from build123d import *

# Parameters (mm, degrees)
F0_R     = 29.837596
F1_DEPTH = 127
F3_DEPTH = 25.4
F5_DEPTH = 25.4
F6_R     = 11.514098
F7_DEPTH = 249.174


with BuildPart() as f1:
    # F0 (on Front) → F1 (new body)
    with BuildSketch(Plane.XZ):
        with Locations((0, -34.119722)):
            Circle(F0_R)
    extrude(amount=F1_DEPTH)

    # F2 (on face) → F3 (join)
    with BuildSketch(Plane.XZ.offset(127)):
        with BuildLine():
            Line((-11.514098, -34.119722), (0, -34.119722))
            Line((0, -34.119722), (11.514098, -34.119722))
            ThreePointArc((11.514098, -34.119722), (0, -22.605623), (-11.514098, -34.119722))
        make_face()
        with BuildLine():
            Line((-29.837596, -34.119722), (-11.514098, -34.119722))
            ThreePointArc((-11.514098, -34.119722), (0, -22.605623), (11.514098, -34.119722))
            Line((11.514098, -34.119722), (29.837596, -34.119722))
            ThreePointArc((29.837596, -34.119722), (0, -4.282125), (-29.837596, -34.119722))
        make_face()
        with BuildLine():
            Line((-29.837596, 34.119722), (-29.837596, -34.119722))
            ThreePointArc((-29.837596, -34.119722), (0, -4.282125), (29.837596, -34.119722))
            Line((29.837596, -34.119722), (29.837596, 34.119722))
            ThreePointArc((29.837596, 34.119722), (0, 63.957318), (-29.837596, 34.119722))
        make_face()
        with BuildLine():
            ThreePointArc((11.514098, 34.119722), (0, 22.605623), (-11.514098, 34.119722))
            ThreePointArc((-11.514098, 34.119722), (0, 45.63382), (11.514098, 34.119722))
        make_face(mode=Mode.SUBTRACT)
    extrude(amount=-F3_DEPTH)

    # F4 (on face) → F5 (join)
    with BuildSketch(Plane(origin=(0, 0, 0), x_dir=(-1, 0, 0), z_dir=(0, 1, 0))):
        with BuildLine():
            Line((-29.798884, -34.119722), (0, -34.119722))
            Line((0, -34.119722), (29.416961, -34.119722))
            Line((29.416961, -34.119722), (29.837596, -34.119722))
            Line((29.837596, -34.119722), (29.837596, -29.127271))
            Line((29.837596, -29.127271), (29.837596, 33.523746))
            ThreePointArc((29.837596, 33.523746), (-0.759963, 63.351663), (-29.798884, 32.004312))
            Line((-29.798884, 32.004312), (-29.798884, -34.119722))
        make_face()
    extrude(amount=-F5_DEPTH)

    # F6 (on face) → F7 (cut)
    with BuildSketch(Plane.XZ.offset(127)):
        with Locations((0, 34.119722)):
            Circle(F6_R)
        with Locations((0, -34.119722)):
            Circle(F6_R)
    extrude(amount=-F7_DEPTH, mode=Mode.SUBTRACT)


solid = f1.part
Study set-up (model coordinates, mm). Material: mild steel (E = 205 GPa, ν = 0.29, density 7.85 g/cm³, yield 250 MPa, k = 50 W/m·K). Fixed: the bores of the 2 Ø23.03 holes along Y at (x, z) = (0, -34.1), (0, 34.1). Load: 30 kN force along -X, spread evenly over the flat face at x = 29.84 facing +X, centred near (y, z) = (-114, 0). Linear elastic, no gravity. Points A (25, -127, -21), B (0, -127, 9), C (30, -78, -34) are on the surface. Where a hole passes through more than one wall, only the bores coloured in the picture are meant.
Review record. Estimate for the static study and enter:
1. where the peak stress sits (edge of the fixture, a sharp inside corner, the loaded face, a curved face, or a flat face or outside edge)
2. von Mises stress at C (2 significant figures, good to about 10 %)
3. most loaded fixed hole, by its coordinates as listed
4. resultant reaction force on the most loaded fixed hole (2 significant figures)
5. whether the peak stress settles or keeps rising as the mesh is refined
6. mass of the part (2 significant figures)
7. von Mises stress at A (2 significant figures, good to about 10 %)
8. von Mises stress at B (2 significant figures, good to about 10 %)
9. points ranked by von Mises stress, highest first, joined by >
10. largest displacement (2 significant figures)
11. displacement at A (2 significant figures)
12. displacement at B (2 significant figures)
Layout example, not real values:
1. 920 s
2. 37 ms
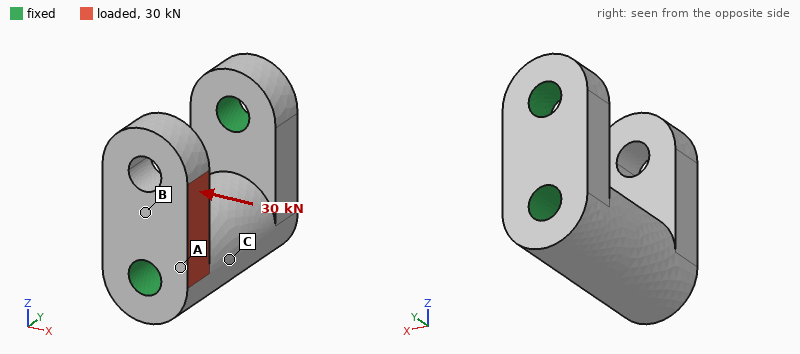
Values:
1. edge of the fixture
2. 9.0 MPa
3. (0, -34.1)
4. 30 kN
5. keeps rising
6. 3.8 kg
7. 36 MPa
8. 23 MPa
9. A > B > C
10. 35 µm
11. 6.8 µm
12. 14 µm
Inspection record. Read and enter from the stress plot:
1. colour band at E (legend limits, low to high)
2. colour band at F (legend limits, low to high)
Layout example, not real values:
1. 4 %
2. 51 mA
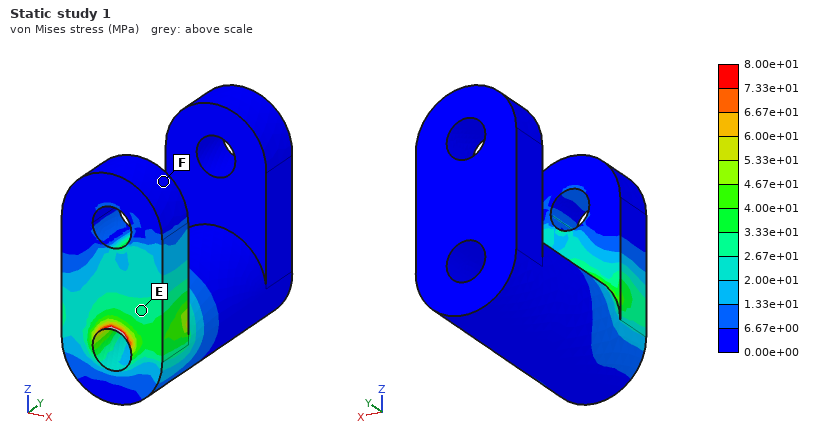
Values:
1. 2.67e+01 to 3.33e+01 MPa
2. 0.00e+00 to 6.67e+00 MPa
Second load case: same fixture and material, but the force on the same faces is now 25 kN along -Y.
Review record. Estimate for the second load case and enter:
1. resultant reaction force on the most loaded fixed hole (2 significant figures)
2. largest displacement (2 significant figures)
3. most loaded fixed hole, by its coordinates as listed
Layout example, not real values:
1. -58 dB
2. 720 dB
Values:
1. 25 kN
2. 57 µm
3. (0, -34.1)
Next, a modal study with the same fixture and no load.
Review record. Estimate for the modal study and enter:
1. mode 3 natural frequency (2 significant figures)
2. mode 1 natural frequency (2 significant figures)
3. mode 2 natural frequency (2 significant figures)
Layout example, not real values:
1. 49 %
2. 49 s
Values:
1. 7600 Hz
2. 3400 Hz
3. 4600 Hz
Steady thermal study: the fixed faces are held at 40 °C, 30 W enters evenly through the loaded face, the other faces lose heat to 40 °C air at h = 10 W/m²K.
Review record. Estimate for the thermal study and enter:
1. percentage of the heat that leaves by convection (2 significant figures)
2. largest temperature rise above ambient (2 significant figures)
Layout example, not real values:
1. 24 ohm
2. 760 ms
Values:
1. 4.1 %
2. 16 K
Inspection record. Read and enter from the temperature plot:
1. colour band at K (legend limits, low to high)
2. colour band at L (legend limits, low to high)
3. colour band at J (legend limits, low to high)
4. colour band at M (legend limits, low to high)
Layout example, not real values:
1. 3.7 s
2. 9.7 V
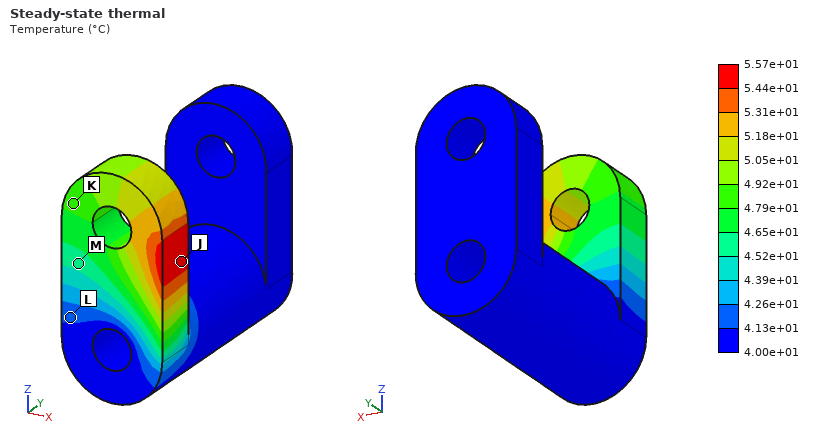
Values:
1. 4.79e+01 to 4.92e+01 °C
2. 4.13e+01 to 4.26e+01 °C
3. 5.44e+01 to 5.57e+01 °C
4. 4.52e+01 to 4.65e+01 °C
